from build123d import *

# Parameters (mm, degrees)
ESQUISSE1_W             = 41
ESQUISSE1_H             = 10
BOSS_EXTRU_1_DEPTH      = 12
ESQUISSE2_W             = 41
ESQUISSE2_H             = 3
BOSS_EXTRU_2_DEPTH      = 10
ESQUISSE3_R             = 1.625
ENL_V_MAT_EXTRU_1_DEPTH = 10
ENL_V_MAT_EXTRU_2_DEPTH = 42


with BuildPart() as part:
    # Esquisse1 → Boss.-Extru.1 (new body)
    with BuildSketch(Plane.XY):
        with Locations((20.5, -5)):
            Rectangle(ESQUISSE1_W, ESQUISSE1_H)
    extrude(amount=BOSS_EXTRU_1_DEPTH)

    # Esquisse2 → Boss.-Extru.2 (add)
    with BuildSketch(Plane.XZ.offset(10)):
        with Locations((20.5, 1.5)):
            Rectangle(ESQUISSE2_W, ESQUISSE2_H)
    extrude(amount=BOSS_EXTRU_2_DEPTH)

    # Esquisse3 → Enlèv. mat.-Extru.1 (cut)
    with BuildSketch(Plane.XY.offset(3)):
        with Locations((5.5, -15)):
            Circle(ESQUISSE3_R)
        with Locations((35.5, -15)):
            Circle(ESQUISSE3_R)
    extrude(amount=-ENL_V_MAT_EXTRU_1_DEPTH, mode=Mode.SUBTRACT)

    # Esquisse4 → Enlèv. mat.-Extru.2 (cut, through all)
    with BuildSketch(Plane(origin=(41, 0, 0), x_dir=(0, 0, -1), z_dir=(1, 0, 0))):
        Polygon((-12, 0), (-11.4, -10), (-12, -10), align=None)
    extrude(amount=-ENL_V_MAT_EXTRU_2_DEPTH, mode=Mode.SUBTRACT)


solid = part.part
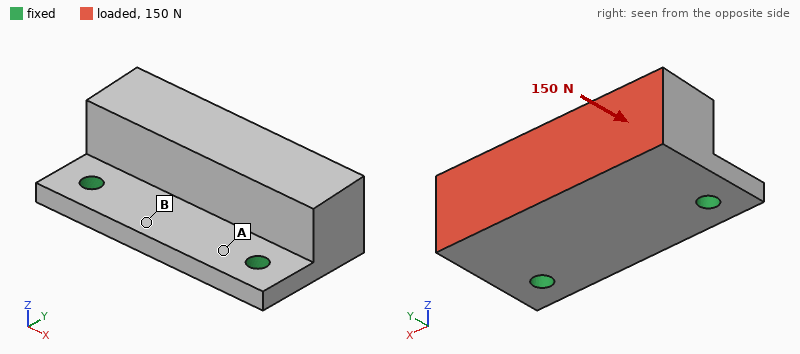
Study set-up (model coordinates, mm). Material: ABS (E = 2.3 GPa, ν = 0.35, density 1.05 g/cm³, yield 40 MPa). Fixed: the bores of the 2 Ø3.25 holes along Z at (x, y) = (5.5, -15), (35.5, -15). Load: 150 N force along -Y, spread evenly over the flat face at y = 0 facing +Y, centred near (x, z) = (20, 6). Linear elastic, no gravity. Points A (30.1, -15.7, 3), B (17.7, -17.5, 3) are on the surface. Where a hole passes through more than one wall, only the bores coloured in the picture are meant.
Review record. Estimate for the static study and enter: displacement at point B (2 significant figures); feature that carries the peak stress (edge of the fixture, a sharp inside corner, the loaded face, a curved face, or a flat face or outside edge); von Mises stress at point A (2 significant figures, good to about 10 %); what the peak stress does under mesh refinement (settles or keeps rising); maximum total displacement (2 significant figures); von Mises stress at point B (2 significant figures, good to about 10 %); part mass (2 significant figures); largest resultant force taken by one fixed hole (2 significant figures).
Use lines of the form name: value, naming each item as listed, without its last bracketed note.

displacement at point B: 0.067 mm
feature that carries the peak stress: edge of the fixture
von Mises stress at point A: 6.6 MPa
what the peak stress does under mesh refinement: keeps rising
maximum total displacement: 0.39 mm
von Mises stress at point B: 2.9 MPa
part mass: 6.3 g
largest resultant force taken by one fixed hole: 77 N
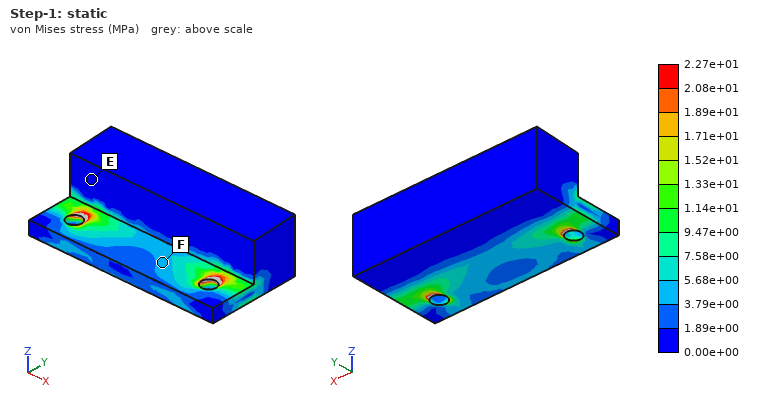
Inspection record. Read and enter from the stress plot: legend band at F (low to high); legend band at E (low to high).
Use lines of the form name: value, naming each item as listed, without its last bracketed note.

legend band at F: 3.79e+00 to 5.68e+00 MPa
legend band at E: 0.00e+00 to 1.89e+00 MPa
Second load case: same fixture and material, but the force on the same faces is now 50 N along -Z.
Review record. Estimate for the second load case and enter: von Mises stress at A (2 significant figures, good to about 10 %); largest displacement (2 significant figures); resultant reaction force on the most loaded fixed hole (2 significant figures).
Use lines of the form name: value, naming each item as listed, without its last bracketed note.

von Mises stress at A: 5.4 MPa
largest displacement: 0.35 mm
resultant reaction force on the most loaded fixed hole: 25 N
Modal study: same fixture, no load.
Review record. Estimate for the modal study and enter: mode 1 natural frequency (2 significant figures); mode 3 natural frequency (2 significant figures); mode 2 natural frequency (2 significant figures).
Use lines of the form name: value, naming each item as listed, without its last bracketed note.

mode 1 natural frequency: 1200 Hz
mode 3 natural frequency: 5600 Hz
mode 2 natural frequency: 3800 Hz
